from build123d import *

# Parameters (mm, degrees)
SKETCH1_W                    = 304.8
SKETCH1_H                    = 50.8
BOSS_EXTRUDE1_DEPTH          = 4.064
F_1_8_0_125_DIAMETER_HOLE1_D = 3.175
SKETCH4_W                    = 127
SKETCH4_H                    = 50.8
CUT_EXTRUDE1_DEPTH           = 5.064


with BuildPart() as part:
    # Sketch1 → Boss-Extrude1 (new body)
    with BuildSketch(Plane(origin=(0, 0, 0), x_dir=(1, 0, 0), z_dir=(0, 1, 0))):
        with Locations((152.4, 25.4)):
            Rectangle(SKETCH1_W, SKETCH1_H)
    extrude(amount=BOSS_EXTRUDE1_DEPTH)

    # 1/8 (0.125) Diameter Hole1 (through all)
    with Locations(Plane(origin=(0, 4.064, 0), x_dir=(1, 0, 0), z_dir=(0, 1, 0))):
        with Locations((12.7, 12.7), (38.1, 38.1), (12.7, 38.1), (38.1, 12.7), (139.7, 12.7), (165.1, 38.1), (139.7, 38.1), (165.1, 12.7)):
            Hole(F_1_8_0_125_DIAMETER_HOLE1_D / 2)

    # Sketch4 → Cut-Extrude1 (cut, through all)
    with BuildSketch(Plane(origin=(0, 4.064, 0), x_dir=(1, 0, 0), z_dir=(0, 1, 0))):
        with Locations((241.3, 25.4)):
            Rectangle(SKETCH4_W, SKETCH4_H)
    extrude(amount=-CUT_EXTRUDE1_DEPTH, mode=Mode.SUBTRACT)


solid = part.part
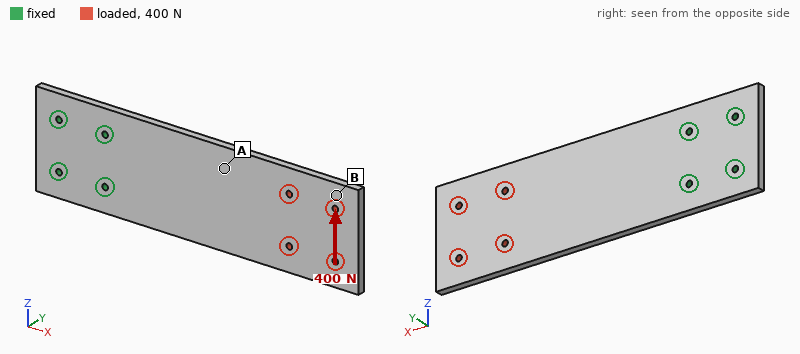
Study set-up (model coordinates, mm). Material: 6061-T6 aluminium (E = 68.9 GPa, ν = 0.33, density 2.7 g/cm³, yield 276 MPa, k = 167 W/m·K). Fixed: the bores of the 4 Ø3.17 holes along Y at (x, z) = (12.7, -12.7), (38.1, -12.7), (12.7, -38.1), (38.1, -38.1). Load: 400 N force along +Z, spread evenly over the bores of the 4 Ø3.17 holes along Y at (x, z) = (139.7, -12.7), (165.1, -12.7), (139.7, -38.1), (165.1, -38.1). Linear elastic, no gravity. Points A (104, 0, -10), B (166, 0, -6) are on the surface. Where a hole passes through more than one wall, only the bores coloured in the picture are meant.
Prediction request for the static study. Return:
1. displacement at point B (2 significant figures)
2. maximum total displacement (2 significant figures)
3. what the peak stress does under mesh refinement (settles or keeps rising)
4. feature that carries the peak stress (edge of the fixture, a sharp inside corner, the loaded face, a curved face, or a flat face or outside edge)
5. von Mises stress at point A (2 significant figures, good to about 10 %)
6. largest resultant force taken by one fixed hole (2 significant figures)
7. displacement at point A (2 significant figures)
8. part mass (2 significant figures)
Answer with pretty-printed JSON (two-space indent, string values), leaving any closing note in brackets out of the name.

{
  "displacement at point B": "0.11 mm",
  "maximum total displacement": "0.12 mm",
  "what the peak stress does under mesh refinement": "keeps rising",
  "feature that carries the peak stress": "edge of the fixture",
  "von Mises stress at point A": "7.4 MPa",
  "largest resultant force taken by one fixed hole": "1.2 kN",
  "displacement at point A": "0.043 mm",
  "part mass": "98 g"
}
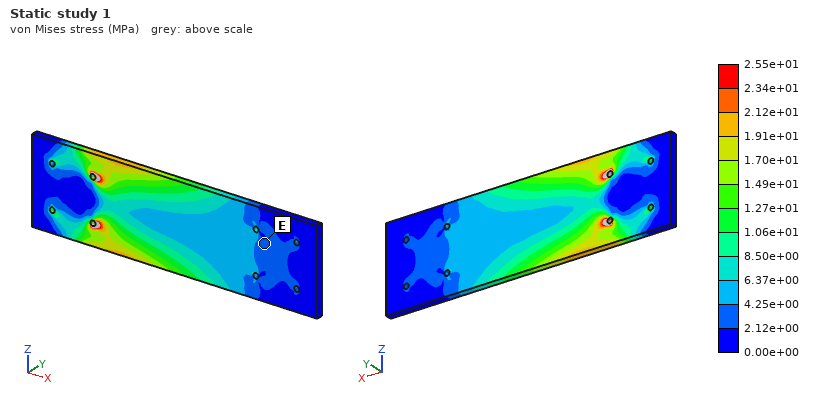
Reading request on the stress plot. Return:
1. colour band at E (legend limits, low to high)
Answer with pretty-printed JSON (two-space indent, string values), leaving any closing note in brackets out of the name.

{
  "colour band at E": "2.12e+00 to 4.25e+00 MPa"
}
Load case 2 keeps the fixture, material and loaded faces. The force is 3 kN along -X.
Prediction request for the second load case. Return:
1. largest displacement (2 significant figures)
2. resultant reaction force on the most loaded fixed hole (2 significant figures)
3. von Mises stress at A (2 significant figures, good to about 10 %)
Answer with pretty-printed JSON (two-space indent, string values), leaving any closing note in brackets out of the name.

{
  "largest displacement": "27 µm",
  "resultant reaction force on the most loaded fixed hole": "1.2 kN",
  "von Mises stress at A": "15 MPa"
}
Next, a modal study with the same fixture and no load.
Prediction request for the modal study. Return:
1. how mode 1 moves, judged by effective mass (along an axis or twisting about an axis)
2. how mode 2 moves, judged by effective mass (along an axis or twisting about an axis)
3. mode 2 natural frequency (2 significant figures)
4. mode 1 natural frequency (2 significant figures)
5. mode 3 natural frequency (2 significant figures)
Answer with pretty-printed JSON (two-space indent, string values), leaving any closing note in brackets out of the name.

{
  "how mode 1 moves, judged by effective mass": "along Y",
  "how mode 2 moves, judged by effective mass": "twisting about X",
  "mode 2 natural frequency": "940 Hz",
  "mode 1 natural frequency": "170 Hz",
  "mode 3 natural frequency": "1100 Hz"
}
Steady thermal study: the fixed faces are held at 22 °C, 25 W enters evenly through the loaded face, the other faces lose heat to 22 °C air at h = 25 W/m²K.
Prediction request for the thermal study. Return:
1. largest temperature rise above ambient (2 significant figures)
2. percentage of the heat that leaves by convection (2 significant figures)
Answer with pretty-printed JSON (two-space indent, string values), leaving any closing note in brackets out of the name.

{
  "largest temperature rise above ambient": "55 K",
  "percentage of the heat that leaves by convection": "47 %"
}
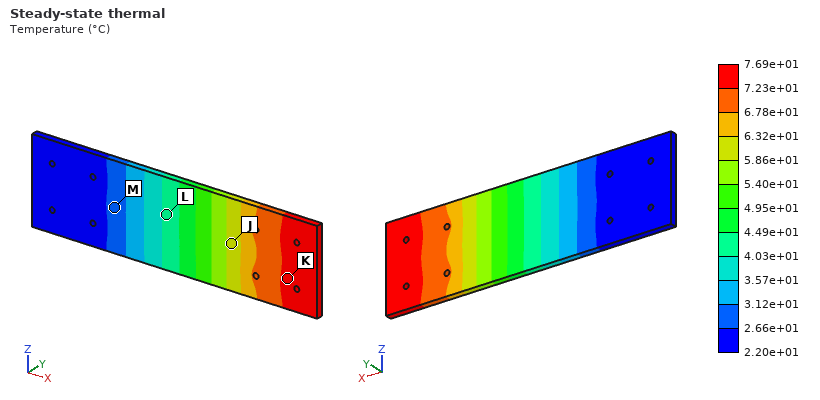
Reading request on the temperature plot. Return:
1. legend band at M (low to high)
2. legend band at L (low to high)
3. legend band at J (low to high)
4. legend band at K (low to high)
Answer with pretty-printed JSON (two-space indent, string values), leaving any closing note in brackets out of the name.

{
  "legend band at M": "2.66e+01 to 3.12e+01 °C",
  "legend band at L": "4.03e+01 to 4.49e+01 °C",
  "legend band at J": "5.86e+01 to 6.32e+01 °C",
  "legend band at K": "7.23e+01 to 7.69e+01 °C"
}
